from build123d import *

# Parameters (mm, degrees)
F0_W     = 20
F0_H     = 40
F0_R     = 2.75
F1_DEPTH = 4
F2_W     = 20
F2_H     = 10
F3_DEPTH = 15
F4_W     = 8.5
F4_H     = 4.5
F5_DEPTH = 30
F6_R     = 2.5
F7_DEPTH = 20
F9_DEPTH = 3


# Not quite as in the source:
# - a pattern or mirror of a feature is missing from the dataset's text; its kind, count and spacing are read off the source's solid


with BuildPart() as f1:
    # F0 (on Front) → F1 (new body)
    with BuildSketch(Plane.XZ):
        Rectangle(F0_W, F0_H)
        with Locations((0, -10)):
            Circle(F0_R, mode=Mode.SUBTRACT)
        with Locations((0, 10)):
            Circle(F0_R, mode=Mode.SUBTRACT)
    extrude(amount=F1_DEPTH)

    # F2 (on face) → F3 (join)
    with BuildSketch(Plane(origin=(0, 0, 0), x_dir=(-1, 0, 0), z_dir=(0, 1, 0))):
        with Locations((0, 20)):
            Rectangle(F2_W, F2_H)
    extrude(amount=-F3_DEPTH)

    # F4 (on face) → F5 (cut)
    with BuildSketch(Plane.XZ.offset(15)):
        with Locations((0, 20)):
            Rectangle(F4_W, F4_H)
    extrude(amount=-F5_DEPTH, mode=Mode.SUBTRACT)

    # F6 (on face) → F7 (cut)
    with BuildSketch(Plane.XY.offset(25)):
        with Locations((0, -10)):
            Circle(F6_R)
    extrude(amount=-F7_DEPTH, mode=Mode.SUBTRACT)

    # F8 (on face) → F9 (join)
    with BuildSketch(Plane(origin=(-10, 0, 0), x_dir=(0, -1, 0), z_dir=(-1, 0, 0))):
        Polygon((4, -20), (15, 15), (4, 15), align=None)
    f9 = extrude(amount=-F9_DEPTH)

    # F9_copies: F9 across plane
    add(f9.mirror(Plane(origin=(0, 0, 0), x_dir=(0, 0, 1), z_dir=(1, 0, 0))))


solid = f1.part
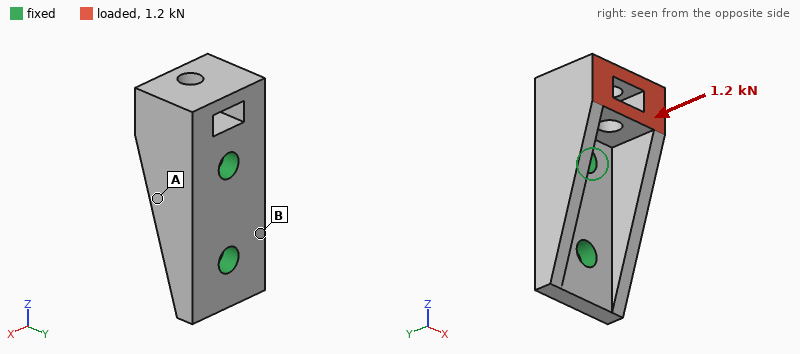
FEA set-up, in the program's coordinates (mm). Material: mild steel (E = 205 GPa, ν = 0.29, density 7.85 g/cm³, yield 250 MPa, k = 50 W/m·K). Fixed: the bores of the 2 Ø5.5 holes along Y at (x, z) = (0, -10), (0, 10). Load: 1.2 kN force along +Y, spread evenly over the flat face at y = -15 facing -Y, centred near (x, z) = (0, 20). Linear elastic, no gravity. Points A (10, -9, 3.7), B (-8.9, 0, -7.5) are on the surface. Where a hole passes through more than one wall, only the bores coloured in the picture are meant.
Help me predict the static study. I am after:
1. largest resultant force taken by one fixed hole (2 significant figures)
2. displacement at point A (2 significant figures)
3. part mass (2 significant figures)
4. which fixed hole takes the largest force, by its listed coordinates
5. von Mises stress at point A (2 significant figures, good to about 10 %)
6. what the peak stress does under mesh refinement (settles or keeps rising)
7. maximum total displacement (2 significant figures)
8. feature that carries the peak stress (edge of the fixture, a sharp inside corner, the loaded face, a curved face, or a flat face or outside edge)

1.5 kN
1.6 µm
48 g
(0, 10)
21 MPa
keeps rising
10 µm
edge of the fixture
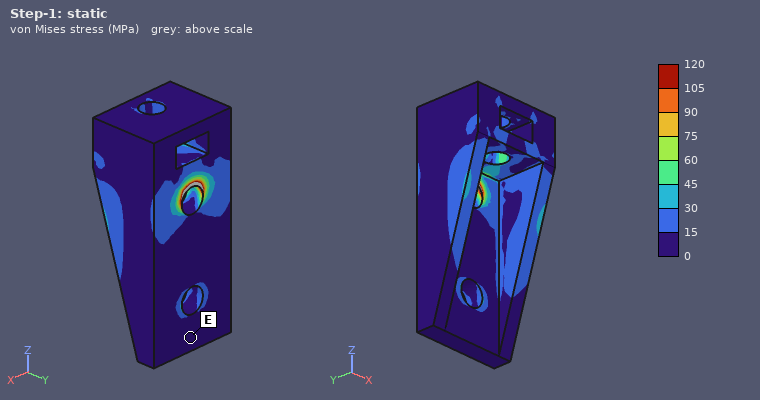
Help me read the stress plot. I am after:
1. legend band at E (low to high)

0 to 15 MPa
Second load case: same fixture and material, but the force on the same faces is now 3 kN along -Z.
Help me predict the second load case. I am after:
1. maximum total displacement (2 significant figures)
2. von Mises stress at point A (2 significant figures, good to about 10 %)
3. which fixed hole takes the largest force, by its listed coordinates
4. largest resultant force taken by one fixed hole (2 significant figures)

35 µm
82 MPa
(0, -10)
2.4 kN
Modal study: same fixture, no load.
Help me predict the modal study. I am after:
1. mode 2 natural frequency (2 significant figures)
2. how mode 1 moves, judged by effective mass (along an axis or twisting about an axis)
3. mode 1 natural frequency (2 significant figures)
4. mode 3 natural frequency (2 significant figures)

14 kHz
along X
11 kHz
21 kHz
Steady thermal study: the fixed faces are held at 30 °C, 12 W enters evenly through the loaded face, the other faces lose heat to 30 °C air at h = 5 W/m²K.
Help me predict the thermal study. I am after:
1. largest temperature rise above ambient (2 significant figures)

37 K
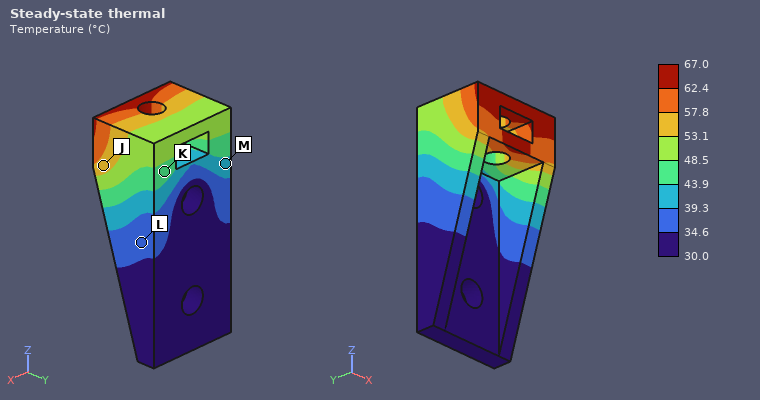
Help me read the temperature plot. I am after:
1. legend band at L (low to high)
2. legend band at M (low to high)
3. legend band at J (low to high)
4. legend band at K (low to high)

34.6 to 39.3 °C
39.3 to 43.9 °C
53.1 to 57.8 °C
43.9 to 48.5 °C
